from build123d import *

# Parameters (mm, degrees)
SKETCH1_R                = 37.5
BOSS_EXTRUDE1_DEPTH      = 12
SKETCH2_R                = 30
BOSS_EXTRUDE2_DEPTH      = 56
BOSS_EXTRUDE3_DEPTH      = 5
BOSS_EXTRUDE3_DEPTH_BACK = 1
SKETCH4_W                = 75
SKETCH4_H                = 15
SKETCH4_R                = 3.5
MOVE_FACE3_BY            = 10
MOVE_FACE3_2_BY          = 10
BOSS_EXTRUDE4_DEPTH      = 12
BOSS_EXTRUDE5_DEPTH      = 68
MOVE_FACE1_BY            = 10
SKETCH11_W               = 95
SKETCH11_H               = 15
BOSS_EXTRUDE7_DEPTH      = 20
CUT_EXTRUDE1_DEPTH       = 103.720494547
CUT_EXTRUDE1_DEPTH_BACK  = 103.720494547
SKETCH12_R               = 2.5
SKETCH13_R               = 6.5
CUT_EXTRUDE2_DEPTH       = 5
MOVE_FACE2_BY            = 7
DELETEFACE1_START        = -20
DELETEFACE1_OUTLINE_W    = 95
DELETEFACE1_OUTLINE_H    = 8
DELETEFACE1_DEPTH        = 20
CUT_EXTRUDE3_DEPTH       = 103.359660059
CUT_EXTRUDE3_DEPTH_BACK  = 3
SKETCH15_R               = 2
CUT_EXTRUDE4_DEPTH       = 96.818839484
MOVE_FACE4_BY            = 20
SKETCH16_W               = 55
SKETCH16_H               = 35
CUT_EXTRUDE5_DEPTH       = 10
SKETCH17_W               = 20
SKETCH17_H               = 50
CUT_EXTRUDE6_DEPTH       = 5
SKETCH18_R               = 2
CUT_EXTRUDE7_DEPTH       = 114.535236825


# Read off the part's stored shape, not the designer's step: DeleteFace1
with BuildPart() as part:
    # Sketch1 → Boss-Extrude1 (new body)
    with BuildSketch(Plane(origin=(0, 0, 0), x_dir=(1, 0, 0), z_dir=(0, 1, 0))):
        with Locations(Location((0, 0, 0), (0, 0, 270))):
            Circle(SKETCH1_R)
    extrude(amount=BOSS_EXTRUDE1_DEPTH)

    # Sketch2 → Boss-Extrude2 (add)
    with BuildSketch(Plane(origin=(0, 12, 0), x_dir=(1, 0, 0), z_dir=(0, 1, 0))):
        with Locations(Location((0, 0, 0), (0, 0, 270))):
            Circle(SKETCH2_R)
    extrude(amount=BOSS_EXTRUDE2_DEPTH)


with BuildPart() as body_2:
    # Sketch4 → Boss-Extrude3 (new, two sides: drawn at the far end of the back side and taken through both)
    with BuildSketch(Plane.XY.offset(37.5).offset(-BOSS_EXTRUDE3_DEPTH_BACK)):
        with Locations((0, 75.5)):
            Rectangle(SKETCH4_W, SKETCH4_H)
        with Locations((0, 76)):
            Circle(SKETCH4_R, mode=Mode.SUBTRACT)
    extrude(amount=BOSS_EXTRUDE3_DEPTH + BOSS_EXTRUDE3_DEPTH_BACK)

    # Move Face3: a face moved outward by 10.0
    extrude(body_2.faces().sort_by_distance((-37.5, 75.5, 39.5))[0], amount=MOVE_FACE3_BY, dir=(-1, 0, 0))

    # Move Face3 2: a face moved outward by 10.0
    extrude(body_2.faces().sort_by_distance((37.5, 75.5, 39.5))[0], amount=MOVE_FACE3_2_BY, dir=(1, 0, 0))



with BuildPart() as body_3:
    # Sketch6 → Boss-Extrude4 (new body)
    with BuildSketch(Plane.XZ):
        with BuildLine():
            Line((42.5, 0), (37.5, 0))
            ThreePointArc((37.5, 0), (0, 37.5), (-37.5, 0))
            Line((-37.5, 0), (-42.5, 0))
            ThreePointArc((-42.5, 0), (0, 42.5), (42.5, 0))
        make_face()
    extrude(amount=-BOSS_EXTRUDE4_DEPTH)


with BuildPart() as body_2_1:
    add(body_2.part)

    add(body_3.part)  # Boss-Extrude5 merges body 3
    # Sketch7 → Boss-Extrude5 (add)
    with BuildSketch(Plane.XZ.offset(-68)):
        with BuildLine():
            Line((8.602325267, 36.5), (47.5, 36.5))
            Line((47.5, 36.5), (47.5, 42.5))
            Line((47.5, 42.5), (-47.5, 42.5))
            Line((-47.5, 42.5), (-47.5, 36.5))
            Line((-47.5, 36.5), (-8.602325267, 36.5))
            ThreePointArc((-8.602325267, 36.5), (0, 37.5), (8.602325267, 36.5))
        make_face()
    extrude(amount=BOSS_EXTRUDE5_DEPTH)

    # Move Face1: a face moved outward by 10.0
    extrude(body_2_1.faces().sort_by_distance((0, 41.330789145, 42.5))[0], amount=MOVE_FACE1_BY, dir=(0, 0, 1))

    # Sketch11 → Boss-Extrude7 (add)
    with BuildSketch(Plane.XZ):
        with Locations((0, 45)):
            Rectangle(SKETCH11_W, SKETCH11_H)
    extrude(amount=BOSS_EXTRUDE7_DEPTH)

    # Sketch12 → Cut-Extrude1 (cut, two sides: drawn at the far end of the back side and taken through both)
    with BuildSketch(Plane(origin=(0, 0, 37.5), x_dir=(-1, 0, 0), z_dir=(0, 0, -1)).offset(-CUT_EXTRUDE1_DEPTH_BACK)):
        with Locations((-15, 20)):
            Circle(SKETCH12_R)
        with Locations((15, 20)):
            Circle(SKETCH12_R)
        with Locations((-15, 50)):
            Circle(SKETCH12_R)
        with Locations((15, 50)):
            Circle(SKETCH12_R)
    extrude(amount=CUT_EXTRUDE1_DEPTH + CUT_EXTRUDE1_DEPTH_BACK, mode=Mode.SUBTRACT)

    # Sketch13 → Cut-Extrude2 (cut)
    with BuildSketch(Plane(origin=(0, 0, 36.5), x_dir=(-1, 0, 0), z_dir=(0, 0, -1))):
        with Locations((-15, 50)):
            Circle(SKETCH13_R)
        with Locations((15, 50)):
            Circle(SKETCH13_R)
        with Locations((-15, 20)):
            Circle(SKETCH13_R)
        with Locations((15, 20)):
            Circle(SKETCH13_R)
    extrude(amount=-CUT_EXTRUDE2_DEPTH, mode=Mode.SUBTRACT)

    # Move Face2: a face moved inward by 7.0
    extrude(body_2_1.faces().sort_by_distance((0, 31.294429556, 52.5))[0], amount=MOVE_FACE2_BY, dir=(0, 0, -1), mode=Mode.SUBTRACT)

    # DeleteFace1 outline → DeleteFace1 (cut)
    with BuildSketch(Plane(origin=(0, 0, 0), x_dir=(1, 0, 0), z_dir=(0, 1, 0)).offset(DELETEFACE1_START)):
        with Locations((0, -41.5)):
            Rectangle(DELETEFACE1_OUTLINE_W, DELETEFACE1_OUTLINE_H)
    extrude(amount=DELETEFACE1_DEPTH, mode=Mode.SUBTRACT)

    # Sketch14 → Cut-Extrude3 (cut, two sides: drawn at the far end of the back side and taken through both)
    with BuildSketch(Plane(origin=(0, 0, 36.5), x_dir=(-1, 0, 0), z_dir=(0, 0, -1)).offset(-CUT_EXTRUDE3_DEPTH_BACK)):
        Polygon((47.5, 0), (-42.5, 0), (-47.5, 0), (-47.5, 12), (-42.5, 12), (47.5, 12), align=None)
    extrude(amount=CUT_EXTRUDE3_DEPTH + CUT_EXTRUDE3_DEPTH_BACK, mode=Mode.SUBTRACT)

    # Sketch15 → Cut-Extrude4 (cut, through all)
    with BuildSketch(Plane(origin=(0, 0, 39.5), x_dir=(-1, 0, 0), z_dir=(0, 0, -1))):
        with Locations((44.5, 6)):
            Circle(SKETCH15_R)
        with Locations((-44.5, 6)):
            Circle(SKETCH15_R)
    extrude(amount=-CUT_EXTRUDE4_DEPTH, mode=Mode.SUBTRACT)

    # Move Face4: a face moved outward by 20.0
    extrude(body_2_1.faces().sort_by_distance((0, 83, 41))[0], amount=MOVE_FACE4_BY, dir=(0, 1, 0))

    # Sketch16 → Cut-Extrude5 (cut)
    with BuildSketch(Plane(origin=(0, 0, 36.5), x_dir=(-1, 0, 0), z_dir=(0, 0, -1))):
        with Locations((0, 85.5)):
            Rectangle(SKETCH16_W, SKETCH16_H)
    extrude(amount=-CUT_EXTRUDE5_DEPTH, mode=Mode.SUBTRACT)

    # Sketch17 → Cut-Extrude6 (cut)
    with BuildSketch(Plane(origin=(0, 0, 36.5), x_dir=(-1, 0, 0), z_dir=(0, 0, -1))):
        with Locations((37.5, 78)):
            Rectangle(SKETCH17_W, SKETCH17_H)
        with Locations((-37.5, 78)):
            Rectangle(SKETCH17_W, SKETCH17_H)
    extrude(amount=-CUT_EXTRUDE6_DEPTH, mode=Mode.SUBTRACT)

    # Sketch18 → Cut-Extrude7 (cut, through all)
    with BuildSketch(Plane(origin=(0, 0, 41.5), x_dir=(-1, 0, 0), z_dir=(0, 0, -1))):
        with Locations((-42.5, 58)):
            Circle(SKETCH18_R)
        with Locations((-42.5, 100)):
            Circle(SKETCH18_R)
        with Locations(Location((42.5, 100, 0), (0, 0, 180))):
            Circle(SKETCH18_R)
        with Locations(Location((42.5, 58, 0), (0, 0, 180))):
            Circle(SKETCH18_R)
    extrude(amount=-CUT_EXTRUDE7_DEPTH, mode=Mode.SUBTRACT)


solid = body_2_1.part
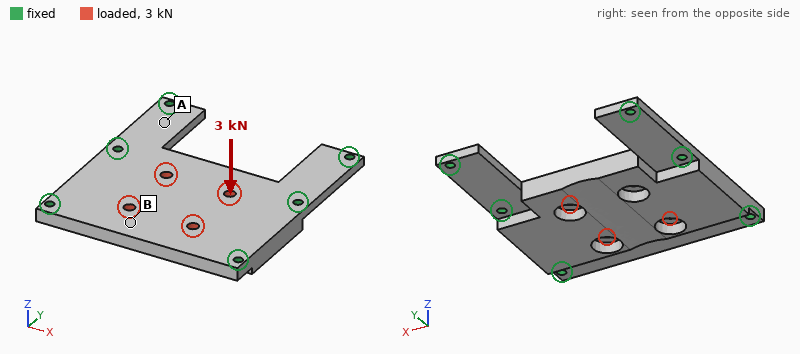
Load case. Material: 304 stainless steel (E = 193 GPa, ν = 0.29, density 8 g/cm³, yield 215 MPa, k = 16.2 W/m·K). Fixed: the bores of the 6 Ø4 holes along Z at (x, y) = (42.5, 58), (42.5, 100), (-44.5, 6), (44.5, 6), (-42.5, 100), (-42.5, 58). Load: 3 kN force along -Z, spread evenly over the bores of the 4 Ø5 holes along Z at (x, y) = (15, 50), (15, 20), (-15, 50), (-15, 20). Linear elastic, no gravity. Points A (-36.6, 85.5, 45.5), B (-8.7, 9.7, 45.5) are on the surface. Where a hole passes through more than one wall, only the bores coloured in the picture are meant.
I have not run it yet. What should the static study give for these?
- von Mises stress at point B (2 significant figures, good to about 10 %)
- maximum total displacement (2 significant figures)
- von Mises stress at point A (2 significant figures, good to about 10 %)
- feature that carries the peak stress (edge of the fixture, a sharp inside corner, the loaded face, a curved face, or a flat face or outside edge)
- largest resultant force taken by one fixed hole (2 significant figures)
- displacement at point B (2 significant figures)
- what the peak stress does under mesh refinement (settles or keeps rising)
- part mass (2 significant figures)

35 MPa
35 µm
14 MPa
edge of the fixture
1.3 kN
33 µm
keeps rising
430 g
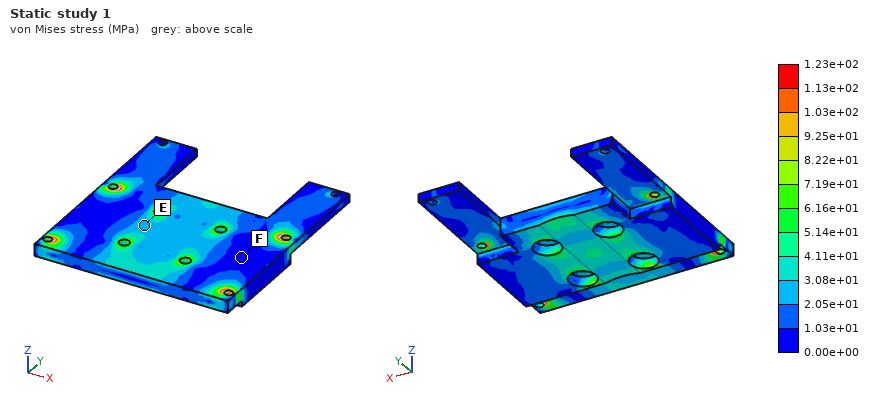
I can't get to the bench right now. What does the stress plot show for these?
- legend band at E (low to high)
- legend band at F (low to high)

2.05e+01 to 3.08e+01 MPa
0.00e+00 to 1.03e+01 MPa
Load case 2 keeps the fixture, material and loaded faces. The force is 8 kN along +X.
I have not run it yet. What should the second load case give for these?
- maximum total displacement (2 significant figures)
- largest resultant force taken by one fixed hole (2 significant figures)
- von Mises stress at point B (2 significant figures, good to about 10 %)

4.5 µm
2.1 kN
9.4 MPa
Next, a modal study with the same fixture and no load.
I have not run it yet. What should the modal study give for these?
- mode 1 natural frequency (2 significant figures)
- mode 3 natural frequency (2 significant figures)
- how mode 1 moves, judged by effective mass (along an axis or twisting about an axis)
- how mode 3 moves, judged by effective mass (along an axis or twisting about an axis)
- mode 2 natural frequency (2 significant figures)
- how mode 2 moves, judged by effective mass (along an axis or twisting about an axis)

3300 Hz
8600 Hz
along Z
twisting about Y
5400 Hz
twisting about X
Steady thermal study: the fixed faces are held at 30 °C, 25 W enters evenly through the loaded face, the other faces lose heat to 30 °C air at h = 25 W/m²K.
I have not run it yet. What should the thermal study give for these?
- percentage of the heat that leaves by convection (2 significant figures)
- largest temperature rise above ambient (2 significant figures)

48 %
59 K
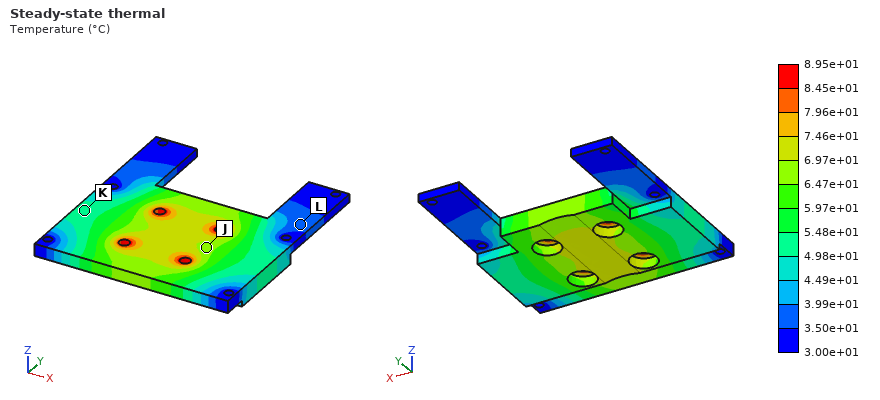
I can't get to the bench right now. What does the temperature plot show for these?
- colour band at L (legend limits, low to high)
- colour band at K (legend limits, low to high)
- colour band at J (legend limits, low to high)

3.50e+01 to 3.99e+01 °C
4.98e+01 to 5.48e+01 °C
6.47e+01 to 6.97e+01 °C
